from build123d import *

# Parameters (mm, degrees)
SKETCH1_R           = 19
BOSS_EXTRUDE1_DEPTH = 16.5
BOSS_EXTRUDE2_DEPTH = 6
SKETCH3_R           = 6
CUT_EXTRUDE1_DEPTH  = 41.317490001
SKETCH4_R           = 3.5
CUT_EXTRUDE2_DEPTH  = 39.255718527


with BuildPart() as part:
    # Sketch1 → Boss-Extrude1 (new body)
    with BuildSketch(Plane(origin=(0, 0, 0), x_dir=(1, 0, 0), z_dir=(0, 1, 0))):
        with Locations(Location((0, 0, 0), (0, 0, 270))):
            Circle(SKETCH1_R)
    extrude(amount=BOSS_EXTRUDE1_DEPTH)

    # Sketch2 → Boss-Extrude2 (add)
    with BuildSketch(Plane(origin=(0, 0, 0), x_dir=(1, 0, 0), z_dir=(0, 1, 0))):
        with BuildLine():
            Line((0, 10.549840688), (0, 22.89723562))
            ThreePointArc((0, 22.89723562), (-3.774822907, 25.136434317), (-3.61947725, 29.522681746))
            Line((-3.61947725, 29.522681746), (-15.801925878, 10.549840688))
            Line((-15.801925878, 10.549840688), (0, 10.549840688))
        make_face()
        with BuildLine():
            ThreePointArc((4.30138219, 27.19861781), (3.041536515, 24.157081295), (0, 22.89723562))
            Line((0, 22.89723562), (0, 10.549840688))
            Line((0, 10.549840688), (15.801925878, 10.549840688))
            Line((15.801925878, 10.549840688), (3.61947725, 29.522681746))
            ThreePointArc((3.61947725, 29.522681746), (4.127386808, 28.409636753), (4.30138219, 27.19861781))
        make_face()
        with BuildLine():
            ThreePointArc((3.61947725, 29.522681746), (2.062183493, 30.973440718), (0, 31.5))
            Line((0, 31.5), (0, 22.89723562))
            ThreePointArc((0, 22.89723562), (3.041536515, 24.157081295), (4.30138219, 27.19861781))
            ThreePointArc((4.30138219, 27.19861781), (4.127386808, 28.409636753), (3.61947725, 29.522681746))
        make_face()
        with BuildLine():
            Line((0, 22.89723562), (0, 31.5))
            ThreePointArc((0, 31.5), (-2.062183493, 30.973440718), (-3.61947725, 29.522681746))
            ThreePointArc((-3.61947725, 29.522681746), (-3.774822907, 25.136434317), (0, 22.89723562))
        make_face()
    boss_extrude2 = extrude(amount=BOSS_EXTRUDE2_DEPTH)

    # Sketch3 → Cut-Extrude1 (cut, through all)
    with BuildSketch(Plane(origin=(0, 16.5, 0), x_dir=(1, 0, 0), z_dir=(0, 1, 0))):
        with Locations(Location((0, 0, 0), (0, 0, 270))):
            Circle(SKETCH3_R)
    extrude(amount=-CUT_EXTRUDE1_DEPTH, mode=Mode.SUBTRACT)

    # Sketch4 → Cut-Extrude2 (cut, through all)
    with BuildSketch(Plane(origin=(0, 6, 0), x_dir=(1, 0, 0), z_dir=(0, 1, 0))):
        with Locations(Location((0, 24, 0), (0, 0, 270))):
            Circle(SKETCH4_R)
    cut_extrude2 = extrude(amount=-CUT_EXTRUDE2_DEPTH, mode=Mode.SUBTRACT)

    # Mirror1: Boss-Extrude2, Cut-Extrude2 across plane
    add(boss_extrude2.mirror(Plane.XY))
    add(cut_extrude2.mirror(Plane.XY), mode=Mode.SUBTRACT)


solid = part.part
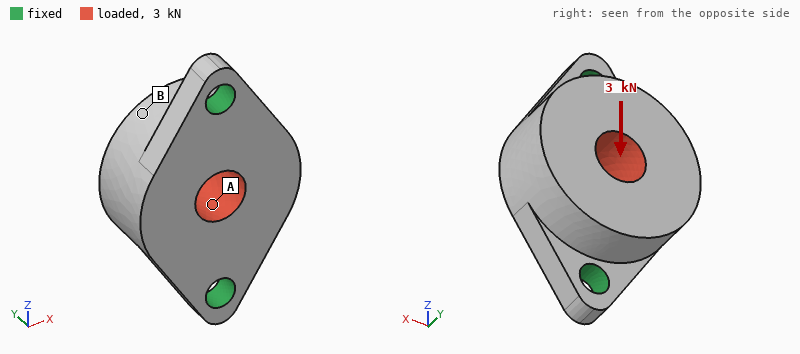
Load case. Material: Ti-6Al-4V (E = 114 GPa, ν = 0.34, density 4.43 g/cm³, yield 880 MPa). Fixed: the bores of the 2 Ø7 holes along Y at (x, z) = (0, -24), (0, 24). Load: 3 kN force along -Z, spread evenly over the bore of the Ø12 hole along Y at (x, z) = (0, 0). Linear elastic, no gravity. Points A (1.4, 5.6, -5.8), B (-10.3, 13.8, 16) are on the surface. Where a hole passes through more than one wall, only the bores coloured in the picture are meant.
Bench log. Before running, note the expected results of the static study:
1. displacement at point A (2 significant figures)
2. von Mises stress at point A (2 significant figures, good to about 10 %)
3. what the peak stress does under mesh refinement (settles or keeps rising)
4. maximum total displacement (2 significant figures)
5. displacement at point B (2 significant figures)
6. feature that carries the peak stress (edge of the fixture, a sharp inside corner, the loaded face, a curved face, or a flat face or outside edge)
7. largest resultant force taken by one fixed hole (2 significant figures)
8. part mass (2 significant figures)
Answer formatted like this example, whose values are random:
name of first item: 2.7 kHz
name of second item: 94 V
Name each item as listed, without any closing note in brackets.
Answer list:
displacement at point A: 1.6 µm
von Mises stress at point A: 6.3 MPa
what the peak stress does under mesh refinement: keeps rising
maximum total displacement: 2.3 µm
displacement at point B: 1.8 µm
feature that carries the peak stress: a sharp inside corner
largest resultant force taken by one fixed hole: 1.5 kN
part mass: 83 g
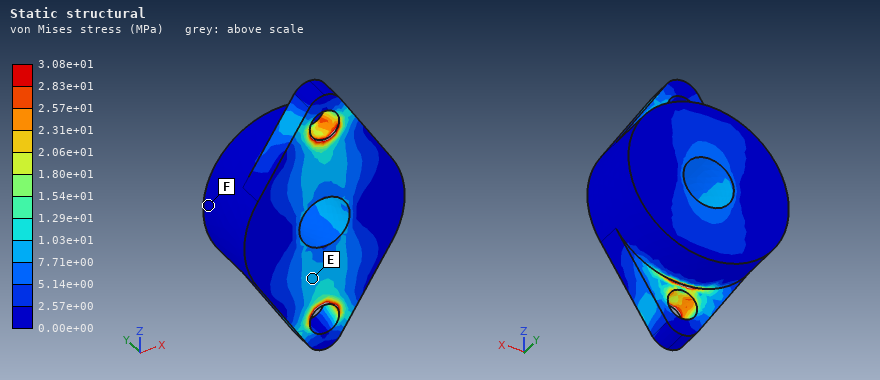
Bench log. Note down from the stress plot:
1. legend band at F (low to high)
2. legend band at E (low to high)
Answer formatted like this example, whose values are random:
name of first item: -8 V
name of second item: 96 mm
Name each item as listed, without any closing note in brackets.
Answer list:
legend band at F: 0.00e+00 to 2.57e+00 MPa
legend band at E: 7.71e+00 to 1.03e+01 MPa
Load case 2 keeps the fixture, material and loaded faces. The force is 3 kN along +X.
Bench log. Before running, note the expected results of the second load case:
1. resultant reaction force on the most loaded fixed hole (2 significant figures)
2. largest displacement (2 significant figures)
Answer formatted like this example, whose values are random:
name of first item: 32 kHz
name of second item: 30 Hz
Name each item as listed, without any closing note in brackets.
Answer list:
resultant reaction force on the most loaded fixed hole: 1.5 kN
largest displacement: 20 µm
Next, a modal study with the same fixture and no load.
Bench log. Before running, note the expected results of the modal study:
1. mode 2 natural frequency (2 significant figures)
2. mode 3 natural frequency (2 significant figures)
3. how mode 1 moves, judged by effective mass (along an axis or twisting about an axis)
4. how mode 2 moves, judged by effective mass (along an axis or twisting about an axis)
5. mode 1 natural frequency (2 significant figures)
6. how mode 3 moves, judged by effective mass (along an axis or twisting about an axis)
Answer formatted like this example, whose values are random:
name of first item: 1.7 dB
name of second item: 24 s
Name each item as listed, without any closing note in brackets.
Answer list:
mode 2 natural frequency: 13 kHz
mode 3 natural frequency: 20 kHz
how mode 1 moves, judged by effective mass: along X
how mode 2 moves, judged by effective mass: along Y
mode 1 natural frequency: 6600 Hz
how mode 3 moves, judged by effective mass: along X
